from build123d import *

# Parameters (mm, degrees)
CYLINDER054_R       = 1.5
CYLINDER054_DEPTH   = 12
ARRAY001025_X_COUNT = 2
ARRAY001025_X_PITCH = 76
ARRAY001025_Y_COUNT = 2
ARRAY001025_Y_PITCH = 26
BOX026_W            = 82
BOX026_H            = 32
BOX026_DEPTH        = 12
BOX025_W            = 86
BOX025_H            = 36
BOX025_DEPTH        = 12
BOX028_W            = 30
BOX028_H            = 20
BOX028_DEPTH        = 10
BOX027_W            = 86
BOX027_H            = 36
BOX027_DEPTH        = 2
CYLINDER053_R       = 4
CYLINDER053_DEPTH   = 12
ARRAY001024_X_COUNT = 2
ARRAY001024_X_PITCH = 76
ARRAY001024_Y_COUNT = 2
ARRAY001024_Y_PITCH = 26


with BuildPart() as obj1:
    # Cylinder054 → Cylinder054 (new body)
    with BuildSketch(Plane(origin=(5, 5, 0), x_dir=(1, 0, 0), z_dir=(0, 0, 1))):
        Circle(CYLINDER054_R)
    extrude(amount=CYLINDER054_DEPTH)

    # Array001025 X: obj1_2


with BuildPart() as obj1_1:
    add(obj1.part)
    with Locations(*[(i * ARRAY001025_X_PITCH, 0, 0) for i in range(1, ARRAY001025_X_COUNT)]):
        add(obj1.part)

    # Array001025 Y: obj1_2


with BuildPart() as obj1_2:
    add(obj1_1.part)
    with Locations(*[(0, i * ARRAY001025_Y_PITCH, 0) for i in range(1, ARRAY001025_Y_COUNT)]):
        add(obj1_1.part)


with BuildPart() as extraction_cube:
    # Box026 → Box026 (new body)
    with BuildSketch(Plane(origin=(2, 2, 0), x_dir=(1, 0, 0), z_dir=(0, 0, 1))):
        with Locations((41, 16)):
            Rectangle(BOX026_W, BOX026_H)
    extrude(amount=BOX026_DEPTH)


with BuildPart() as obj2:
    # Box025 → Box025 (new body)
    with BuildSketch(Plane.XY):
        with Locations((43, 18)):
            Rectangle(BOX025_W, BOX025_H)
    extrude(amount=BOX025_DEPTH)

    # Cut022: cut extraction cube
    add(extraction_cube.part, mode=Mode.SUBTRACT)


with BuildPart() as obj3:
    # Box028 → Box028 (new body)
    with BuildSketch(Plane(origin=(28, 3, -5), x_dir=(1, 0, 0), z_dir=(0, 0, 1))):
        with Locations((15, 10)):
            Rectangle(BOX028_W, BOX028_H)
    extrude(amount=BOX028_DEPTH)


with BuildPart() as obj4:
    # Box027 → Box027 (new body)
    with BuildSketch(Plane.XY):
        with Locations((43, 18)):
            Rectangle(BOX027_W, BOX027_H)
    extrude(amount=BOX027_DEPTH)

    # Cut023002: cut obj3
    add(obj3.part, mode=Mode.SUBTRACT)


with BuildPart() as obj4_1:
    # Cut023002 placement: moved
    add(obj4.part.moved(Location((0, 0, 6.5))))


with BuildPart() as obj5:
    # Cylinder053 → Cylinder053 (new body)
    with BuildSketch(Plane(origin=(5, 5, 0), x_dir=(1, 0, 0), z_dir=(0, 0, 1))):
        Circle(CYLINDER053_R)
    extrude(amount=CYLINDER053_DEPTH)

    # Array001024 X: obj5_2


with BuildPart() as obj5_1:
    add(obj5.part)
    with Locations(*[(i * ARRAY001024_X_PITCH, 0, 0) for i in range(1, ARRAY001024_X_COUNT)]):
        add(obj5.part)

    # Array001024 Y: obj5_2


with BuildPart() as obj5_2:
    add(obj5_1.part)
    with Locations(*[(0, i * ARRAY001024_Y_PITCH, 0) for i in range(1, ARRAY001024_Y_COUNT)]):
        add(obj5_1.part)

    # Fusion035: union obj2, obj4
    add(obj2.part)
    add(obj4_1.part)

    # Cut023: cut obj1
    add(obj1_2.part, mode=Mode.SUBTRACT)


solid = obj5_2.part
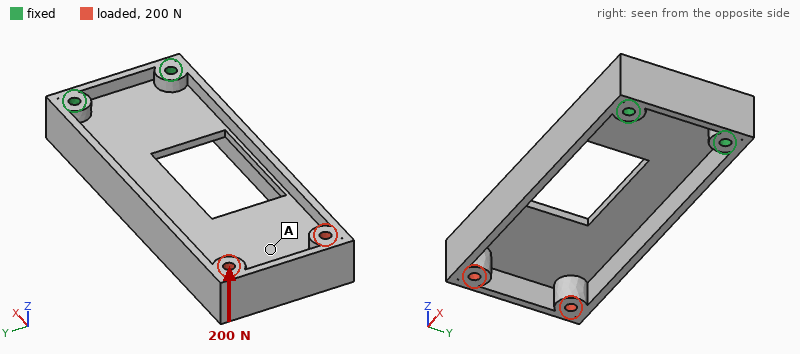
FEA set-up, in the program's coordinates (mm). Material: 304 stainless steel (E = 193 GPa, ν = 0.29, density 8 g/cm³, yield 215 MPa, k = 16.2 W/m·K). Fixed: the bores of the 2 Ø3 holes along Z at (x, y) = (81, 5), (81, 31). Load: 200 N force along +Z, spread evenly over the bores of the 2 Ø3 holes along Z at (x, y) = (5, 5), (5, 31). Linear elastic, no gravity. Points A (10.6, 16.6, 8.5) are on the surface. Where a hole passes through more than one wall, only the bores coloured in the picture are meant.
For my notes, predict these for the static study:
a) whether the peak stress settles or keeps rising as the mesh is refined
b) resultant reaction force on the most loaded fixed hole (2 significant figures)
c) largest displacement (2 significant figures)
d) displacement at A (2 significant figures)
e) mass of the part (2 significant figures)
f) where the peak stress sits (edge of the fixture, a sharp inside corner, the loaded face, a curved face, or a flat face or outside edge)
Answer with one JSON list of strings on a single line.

["keeps rising", "110 N", "0.28 mm", "0.22 mm", "89 g", "a sharp inside corner"]
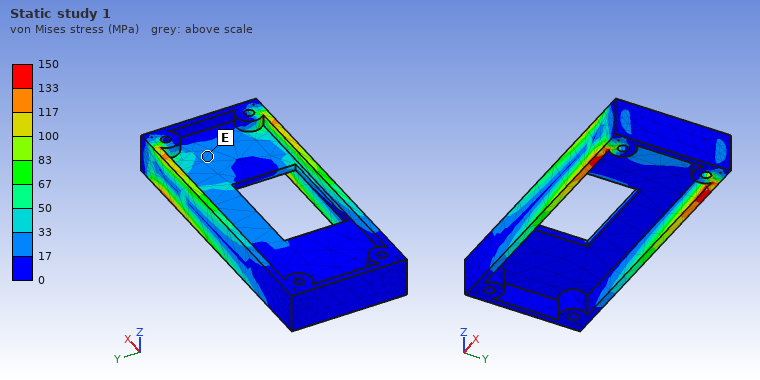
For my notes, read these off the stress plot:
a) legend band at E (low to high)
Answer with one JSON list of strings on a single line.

["17 to 33 MPa"]
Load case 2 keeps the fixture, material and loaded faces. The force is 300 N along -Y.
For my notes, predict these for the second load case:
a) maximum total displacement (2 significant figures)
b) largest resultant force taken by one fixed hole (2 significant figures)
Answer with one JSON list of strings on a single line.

["65 µm", "800 N"]
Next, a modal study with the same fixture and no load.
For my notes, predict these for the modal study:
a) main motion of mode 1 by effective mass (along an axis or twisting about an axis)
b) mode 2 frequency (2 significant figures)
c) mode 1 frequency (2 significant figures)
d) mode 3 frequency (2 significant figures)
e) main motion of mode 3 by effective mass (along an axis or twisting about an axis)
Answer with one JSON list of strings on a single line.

["along Z", "1400 Hz", "800 Hz", "2400 Hz", "along Y"]
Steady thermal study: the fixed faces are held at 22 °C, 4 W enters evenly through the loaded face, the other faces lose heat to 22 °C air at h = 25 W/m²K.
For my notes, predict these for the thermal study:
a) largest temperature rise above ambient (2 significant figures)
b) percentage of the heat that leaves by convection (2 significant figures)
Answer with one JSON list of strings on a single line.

["43 K", "95 %"]
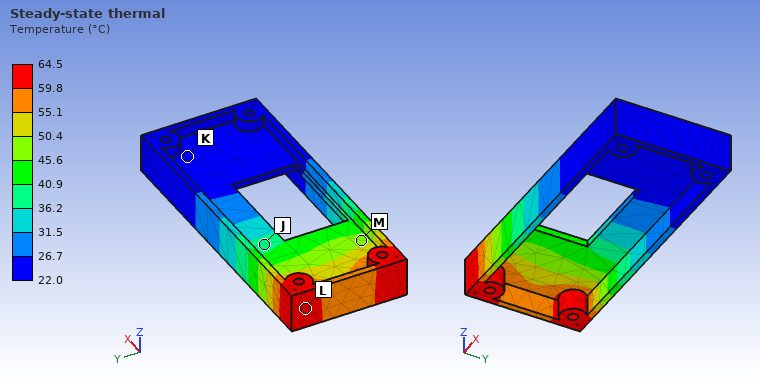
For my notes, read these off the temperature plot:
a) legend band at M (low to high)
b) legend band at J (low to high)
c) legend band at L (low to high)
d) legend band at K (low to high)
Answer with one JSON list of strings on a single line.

["45.6 to 50.4 °C", "36.2 to 40.9 °C", "59.8 to 64.5 °C", "22.0 to 26.7 °C"]
